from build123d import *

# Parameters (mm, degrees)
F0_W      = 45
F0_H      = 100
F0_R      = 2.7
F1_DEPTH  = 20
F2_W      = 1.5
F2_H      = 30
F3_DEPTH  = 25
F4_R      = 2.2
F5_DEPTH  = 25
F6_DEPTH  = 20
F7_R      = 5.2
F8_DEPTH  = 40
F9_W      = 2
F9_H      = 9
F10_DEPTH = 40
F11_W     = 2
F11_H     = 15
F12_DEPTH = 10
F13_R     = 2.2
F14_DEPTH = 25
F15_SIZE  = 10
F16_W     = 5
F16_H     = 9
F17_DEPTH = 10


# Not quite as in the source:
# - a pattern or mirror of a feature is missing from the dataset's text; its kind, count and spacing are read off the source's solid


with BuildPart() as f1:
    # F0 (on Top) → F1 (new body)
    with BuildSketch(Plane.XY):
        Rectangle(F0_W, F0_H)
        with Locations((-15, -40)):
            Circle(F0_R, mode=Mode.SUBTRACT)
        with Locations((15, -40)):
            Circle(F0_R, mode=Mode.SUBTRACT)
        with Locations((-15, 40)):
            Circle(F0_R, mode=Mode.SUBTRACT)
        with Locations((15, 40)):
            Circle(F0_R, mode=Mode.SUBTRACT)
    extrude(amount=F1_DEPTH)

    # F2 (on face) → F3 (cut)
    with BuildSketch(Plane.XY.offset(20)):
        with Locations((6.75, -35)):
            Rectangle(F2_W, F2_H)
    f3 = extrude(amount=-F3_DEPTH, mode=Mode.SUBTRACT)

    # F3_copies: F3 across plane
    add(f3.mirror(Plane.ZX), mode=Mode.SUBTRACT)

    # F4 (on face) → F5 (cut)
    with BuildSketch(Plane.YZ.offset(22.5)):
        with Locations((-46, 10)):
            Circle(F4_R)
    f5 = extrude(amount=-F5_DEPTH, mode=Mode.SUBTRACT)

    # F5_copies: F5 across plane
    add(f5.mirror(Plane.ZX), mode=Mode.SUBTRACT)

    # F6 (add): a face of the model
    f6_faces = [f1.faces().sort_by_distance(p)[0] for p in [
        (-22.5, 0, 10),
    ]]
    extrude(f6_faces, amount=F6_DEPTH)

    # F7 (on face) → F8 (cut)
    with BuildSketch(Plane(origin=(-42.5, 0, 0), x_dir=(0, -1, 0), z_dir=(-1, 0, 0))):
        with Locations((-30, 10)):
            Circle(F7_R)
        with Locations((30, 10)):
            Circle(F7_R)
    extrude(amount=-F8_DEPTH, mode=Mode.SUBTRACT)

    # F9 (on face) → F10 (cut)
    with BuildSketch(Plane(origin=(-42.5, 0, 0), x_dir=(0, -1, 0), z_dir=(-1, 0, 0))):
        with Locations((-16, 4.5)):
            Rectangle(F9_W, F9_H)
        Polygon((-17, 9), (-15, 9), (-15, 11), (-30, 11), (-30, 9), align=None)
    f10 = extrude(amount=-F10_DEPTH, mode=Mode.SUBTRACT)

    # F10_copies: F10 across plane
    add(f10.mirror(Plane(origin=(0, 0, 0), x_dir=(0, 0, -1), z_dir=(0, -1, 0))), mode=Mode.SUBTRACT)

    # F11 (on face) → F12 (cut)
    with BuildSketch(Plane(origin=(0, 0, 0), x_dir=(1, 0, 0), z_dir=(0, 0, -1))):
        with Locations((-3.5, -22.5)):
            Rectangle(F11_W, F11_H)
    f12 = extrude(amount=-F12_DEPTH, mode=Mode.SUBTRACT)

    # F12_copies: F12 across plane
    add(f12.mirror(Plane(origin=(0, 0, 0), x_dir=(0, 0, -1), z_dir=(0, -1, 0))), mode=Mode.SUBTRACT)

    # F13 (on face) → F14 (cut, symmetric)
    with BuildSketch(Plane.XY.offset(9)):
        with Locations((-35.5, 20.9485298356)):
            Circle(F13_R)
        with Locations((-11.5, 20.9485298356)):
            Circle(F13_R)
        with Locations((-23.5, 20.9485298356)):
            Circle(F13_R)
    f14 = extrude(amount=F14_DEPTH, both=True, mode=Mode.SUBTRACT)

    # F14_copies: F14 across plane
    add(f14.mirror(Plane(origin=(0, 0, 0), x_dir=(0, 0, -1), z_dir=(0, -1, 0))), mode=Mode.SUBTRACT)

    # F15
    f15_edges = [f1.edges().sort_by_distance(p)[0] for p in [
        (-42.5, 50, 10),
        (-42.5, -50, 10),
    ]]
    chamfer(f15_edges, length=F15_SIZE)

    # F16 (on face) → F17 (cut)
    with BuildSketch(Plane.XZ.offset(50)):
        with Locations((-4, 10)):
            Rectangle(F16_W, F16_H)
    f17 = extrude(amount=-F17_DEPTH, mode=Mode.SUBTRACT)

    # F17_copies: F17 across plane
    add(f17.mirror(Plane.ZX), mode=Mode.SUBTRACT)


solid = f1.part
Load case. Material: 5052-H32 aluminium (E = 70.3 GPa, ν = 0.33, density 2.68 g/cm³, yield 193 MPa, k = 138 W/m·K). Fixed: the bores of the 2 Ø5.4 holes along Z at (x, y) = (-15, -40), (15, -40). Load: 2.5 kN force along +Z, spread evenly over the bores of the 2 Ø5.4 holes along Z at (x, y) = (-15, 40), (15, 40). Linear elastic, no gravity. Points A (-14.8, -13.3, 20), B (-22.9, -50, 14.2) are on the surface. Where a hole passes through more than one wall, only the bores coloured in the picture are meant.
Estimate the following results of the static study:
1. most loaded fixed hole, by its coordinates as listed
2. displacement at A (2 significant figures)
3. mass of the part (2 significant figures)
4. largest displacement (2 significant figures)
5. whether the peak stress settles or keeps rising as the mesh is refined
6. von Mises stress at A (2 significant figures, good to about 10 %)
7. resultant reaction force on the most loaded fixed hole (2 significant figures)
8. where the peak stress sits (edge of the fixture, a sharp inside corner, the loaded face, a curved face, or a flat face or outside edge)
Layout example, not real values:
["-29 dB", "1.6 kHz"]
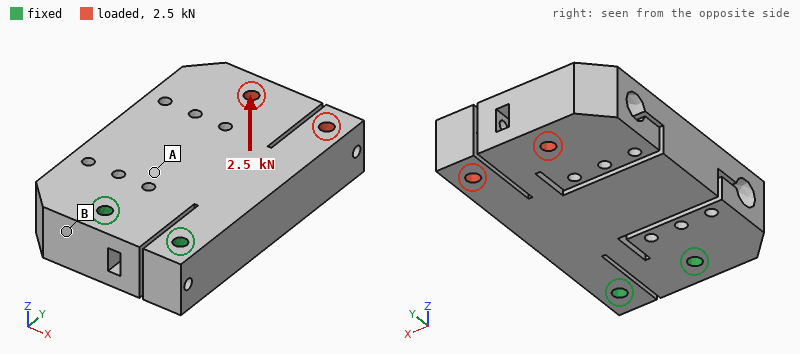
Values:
["(15, -40)", "0.084 mm", "300 g", "0.47 mm", "keeps rising", "29 MPa", "1.8 kN", "edge of the fixture"]
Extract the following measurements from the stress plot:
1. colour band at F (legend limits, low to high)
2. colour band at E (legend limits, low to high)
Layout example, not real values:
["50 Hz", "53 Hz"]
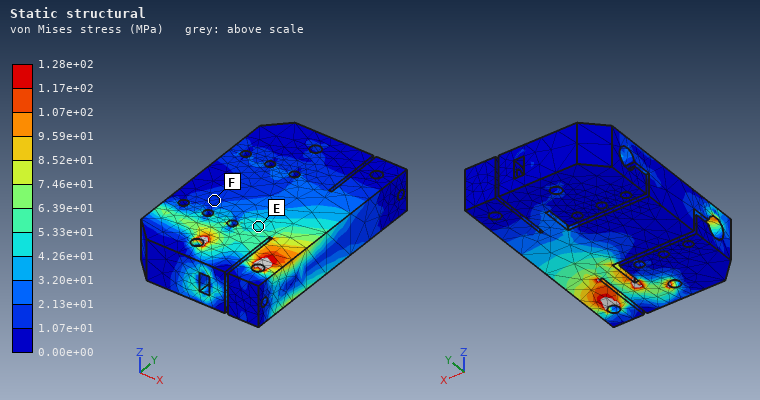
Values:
["1.07e+01 to 2.13e+01 MPa", "4.26e+01 to 5.33e+01 MPa"]
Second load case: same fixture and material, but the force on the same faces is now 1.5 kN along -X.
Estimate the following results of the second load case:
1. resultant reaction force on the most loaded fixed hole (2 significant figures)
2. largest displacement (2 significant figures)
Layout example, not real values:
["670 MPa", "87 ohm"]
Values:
["3.4 kN", "77 µm"]
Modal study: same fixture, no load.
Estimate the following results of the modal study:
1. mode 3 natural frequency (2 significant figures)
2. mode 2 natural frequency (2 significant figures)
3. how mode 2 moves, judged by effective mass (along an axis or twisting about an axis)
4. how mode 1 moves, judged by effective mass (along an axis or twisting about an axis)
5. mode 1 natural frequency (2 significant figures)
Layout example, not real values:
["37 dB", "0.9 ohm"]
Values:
["3600 Hz", "2900 Hz", "along X", "along Z", "1300 Hz"]
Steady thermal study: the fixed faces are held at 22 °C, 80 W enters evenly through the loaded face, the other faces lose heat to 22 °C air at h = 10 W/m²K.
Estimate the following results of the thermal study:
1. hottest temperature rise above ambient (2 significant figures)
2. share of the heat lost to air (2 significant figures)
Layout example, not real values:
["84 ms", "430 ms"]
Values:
["64 K", "10.0 %"]
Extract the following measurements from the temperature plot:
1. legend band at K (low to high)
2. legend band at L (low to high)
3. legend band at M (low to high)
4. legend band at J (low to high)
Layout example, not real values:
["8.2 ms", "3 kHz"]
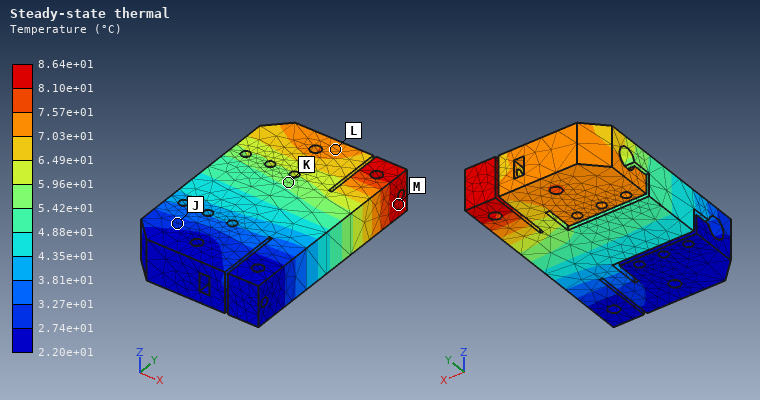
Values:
["5.42e+01 to 5.96e+01 °C", "7.03e+01 to 7.57e+01 °C", "8.10e+01 to 8.64e+01 °C", "2.74e+01 to 3.27e+01 °C"]
